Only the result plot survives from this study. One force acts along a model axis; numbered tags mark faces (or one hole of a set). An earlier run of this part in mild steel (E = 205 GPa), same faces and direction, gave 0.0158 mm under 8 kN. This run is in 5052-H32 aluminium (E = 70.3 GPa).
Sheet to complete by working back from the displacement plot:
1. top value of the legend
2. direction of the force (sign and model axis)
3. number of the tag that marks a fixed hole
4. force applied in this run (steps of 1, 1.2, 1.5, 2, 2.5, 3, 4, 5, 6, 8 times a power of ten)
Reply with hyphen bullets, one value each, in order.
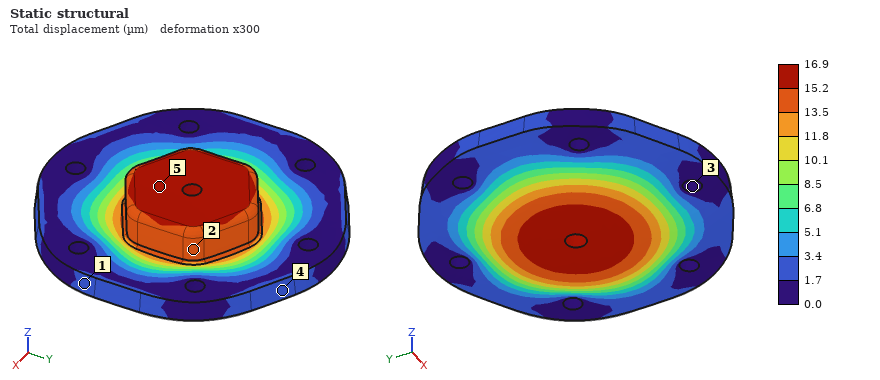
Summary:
- 16.9 µm
- -Z
- 3
- 3 kN
